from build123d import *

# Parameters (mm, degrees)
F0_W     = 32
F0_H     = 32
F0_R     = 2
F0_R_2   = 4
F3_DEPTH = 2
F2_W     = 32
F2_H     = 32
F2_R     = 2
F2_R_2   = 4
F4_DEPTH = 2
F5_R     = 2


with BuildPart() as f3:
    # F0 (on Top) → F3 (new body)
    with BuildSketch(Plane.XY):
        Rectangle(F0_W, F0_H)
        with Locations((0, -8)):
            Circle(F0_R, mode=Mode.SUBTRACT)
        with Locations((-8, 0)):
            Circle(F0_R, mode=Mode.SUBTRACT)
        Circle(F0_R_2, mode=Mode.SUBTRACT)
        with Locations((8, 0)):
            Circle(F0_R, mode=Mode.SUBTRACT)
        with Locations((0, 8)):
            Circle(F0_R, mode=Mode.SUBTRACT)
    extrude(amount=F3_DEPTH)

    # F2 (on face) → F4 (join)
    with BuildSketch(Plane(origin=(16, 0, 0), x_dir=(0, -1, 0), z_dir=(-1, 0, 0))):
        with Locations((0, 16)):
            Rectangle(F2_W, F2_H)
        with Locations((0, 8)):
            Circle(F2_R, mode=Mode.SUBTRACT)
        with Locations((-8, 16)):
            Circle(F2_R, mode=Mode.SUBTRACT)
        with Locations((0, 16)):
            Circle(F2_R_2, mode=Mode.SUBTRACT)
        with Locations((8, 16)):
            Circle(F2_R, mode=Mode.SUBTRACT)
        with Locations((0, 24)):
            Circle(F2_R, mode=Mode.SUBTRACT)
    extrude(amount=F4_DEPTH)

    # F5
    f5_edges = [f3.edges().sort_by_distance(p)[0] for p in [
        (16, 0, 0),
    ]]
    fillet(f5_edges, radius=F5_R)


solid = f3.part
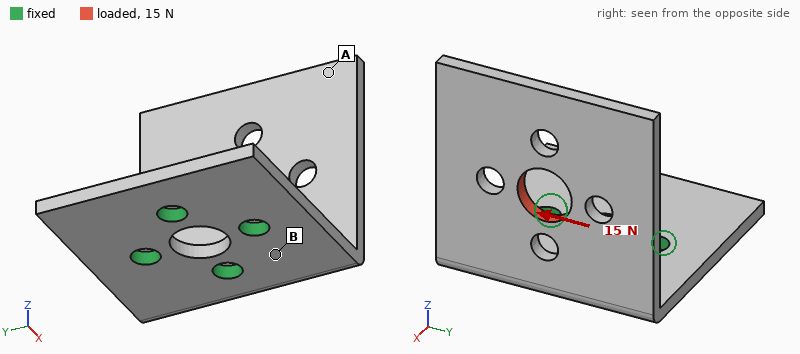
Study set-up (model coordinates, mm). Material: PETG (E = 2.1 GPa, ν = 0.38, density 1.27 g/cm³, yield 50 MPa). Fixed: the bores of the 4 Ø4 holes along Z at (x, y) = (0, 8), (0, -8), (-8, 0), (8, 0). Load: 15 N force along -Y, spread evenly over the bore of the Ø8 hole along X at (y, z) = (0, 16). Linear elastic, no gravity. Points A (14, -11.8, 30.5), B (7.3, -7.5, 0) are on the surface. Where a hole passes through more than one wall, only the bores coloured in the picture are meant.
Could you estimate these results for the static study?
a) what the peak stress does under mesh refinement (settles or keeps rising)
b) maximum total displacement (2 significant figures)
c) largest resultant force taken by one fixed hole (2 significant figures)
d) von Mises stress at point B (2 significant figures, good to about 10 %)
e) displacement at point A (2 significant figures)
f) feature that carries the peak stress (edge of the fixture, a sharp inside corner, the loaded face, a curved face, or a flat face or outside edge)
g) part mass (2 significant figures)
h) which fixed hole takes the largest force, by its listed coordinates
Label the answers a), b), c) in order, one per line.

a) keeps rising
b) 0.55 mm
c) 14 N
d) 4.0 MPa
e) 0.50 mm
f) edge of the fixture
g) 4.5 g
h) (8, 0)
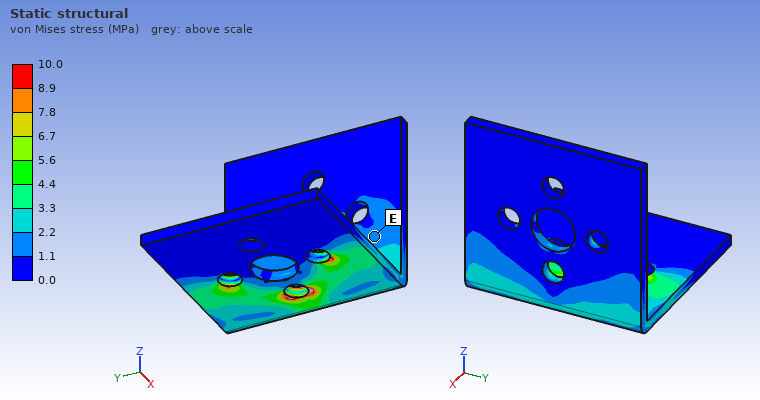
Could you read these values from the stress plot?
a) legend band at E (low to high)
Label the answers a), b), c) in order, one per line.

a) 1.1 to 2.2 MPa
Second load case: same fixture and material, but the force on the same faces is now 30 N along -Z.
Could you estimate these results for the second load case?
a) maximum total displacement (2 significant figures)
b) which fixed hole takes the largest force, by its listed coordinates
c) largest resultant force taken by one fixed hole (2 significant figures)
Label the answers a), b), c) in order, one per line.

a) 0.51 mm
b) (8, 0)
c) 34 N
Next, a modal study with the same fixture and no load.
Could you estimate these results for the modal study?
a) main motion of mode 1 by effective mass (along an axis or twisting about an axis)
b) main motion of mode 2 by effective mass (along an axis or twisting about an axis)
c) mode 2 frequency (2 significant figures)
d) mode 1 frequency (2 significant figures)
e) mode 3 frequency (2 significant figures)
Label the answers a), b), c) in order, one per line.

a) along X
b) along Y
c) 590 Hz
d) 330 Hz
e) 920 Hz
